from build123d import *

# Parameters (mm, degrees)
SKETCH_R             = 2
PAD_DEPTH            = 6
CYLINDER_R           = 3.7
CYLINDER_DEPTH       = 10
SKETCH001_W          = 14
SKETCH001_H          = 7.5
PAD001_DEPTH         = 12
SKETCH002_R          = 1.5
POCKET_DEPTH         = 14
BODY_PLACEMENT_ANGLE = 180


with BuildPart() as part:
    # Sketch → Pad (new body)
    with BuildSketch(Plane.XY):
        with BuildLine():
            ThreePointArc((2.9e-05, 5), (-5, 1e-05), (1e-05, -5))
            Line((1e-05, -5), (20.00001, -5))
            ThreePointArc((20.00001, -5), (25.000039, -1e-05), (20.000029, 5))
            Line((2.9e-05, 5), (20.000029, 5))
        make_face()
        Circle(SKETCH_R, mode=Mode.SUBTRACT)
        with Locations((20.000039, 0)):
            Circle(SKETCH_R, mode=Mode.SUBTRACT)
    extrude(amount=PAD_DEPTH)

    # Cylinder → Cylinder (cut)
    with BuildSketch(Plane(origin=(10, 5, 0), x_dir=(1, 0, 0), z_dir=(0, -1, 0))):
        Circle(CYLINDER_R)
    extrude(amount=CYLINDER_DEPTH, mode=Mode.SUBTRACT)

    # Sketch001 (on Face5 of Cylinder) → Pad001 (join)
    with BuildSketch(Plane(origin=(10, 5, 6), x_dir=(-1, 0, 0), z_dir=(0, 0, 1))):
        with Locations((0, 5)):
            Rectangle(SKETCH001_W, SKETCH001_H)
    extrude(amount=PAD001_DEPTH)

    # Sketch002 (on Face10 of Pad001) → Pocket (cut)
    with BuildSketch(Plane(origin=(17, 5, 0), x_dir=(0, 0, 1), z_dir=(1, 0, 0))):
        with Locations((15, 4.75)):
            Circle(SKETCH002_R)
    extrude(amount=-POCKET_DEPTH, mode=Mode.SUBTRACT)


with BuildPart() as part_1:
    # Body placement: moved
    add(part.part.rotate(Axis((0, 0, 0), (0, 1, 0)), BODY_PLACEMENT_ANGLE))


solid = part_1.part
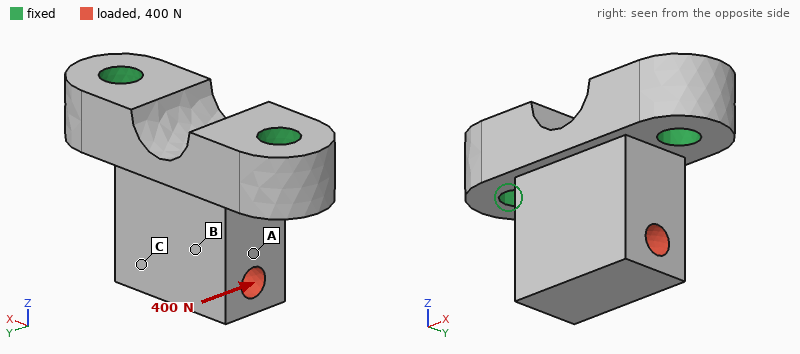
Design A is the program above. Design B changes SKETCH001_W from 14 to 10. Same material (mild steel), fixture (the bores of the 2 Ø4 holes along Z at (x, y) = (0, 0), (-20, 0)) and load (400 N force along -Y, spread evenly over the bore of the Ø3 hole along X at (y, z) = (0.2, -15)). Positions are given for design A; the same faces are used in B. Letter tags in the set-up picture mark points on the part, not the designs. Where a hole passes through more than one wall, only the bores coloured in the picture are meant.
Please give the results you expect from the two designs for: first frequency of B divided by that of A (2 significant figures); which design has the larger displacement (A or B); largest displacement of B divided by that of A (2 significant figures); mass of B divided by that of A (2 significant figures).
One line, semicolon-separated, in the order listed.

0.96; B; 1.5; 0.87
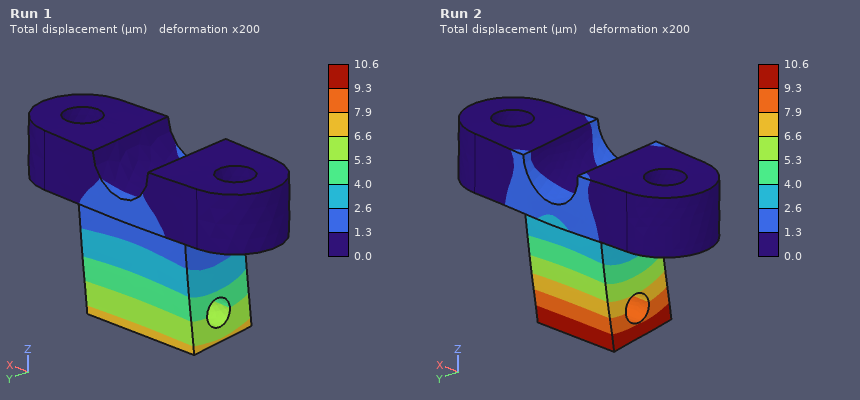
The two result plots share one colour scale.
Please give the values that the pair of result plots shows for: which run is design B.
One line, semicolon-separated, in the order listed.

Run 2
